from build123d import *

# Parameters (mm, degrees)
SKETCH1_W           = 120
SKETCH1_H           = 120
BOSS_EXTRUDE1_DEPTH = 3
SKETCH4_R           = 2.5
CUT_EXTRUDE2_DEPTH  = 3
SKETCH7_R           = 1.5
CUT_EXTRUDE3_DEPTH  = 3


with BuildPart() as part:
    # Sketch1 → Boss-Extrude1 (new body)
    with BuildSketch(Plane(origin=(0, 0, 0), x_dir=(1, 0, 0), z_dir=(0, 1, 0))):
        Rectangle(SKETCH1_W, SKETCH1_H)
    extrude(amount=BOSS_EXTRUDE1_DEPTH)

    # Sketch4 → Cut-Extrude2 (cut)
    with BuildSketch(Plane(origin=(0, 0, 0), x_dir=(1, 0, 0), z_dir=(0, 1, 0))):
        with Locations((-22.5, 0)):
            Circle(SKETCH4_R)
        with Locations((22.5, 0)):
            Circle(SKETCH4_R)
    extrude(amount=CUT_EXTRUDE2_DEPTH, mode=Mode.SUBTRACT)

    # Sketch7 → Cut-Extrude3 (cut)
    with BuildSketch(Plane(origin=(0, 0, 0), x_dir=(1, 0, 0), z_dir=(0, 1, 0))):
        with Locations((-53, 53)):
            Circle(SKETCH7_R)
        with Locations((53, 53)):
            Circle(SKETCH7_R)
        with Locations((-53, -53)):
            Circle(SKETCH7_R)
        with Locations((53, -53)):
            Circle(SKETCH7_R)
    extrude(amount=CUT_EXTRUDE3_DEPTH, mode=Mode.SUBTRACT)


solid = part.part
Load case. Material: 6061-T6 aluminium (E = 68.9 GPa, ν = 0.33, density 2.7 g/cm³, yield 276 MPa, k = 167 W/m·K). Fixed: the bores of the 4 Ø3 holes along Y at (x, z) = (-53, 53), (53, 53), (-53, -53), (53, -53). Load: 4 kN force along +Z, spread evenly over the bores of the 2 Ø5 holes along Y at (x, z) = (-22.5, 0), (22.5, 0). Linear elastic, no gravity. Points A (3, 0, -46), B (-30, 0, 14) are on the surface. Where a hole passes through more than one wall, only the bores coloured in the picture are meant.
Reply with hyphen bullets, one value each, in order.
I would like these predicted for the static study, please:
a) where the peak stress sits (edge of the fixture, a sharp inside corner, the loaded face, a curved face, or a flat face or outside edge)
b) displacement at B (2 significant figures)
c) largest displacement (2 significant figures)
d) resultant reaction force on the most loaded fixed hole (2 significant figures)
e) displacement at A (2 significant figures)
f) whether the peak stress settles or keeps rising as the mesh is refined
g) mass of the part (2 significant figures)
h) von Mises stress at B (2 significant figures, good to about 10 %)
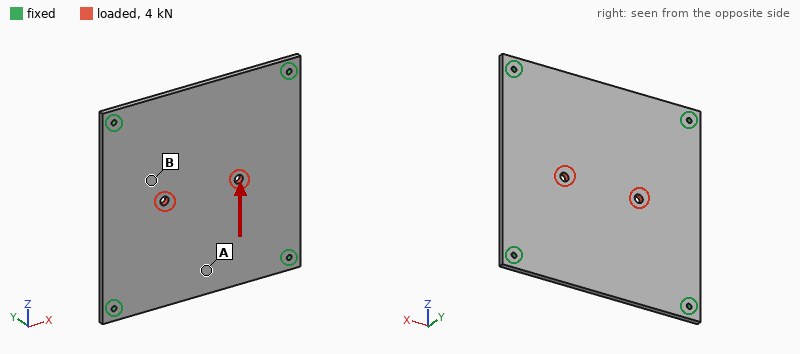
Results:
- edge of the fixture
- 12 µm
- 18 µm
- 1.1 kN
- 13 µm
- keeps rising
- 120 g
- 15 MPa
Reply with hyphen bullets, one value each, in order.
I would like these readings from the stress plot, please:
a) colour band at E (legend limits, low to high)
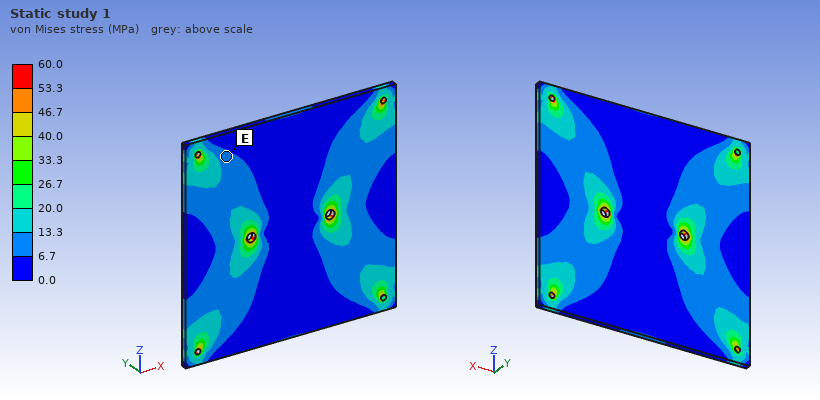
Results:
- 6.7 to 13.3 MPa
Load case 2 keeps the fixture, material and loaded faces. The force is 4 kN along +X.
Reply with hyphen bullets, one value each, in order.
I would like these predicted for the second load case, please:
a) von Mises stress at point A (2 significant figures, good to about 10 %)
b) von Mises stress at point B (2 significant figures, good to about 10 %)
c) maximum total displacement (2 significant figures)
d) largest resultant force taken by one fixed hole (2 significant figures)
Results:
- 6.8 MPa
- 12 MPa
- 22 µm
- 1.1 kN
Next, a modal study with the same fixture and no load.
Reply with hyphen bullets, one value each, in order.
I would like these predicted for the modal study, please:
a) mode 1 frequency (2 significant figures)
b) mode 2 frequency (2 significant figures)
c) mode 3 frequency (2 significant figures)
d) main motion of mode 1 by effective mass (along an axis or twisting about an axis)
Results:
- 830 Hz
- 1500 Hz
- 1500 Hz
- along Y
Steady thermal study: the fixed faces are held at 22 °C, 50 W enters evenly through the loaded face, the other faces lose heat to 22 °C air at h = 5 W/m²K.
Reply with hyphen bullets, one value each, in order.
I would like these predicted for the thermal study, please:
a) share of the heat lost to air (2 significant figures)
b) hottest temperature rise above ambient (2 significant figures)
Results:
- 7.1 %
- 48 K
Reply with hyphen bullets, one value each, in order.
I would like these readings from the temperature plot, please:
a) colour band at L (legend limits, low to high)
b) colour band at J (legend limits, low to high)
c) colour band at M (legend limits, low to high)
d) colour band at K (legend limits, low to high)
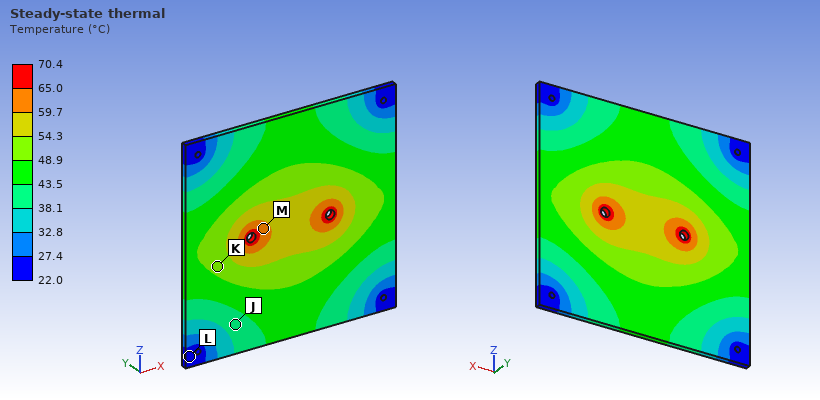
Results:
- 22.0 to 27.4 °C
- 38.1 to 43.5 °C
- 59.7 to 65.0 °C
- 48.9 to 54.3 °C
